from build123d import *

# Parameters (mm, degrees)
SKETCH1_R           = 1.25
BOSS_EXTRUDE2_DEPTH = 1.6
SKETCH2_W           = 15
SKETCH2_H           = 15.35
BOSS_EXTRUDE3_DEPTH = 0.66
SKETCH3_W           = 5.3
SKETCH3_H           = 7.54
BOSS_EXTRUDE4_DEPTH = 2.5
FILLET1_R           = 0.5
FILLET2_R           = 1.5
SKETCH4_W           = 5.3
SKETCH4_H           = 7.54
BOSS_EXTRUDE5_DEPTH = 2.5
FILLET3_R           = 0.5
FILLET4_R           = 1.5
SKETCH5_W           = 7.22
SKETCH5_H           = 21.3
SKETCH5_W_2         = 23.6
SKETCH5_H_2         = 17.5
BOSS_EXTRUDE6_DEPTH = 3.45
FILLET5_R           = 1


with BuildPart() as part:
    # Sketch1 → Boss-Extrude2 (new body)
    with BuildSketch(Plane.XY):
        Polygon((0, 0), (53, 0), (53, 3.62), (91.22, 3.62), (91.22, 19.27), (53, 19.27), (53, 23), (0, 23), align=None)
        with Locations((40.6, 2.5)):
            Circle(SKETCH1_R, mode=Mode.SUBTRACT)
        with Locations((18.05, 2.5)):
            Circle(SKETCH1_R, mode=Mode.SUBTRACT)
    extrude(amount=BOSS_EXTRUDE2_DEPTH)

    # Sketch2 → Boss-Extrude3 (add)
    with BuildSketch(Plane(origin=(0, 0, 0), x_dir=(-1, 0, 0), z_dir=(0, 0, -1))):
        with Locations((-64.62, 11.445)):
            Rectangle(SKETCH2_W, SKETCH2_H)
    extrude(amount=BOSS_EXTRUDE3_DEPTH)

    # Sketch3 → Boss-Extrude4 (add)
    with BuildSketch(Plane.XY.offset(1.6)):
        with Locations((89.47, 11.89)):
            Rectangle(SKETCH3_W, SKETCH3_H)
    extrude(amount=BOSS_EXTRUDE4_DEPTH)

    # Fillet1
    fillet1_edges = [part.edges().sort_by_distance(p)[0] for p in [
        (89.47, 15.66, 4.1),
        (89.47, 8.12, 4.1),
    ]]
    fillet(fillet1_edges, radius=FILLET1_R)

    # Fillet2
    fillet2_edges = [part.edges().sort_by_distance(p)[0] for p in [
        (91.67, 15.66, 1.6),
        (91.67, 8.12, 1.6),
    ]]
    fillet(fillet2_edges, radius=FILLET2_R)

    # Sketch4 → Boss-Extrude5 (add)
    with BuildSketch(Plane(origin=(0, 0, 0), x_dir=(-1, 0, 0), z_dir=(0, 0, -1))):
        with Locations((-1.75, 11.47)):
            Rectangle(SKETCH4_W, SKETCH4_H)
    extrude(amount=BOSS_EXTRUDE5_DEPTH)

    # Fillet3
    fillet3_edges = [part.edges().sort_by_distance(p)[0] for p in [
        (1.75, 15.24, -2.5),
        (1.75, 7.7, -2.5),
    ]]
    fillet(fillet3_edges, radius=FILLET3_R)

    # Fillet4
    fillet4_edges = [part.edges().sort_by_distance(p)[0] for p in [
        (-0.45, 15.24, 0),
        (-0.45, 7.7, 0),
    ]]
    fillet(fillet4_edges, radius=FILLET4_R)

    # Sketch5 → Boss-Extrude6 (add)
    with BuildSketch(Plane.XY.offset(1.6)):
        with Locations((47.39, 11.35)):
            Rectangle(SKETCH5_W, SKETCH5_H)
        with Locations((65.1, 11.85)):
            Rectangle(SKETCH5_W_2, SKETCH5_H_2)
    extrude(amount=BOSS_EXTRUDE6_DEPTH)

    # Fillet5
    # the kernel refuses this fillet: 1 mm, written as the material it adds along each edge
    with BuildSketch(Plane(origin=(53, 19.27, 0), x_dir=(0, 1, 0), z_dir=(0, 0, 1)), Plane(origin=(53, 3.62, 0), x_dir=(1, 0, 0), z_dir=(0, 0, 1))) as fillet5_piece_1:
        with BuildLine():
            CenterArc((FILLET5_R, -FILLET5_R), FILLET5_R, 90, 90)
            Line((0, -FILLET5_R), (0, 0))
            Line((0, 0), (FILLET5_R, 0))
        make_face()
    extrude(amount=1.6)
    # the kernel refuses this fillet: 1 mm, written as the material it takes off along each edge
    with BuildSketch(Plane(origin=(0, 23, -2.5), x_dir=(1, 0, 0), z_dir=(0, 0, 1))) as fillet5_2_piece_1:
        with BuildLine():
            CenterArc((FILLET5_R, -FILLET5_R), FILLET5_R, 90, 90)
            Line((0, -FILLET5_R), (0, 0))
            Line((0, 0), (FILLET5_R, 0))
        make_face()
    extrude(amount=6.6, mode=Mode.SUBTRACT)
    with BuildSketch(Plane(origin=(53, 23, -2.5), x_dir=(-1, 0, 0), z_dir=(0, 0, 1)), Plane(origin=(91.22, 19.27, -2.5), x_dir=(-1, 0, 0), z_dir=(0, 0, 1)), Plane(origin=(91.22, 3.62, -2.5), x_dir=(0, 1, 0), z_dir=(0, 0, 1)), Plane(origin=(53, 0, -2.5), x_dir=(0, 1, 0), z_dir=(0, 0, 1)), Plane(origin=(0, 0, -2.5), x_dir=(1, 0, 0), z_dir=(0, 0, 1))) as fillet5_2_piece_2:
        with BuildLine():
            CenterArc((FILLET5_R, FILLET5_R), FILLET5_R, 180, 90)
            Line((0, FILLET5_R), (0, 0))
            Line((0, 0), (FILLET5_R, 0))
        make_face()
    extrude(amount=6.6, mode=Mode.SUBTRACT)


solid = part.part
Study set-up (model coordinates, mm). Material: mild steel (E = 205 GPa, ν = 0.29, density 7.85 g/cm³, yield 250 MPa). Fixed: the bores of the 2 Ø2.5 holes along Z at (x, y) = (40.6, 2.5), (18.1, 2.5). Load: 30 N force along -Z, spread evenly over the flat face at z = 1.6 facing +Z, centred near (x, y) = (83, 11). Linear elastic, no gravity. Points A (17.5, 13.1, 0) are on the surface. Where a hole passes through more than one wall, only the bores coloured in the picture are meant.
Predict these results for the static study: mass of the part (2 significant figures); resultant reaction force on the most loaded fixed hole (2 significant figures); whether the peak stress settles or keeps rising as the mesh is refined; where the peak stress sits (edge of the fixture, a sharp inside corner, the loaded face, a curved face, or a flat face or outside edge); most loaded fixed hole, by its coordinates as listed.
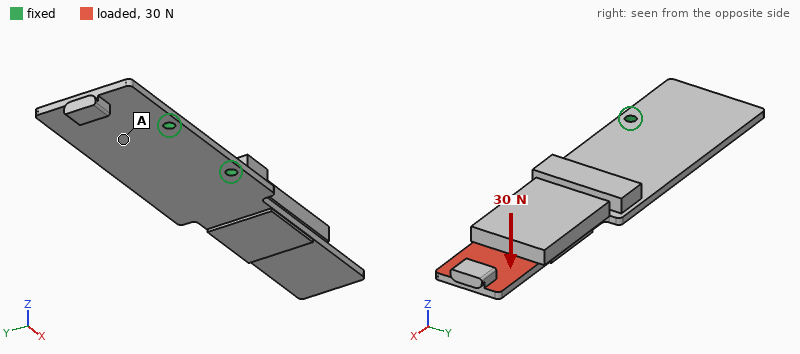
41 g
52 N
keeps rising
edge of the fixture
(40.6, 2.5)
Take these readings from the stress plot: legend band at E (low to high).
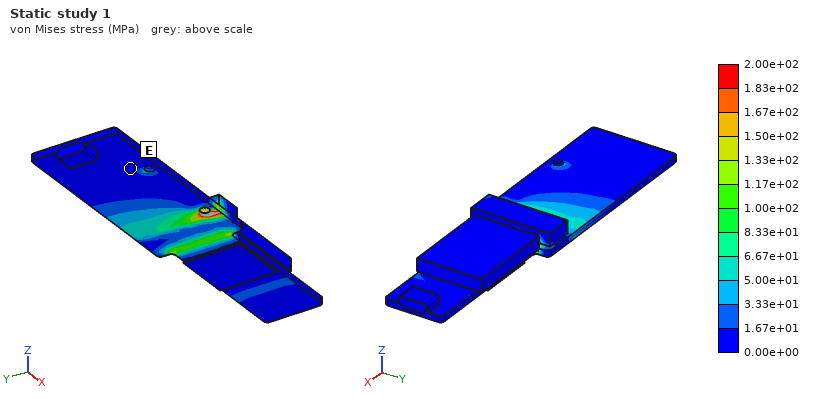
0.00e+00 to 1.67e+01 MPa
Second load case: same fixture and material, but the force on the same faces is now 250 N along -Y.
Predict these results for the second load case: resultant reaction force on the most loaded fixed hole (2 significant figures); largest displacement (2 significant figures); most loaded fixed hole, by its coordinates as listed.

740 N
58 µm
(40.6, 2.5)
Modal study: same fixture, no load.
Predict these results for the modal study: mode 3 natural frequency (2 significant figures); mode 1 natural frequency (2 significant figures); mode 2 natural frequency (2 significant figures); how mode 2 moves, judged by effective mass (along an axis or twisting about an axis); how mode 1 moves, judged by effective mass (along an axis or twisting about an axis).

2400 Hz
520 Hz
2200 Hz
along Z
along Z
